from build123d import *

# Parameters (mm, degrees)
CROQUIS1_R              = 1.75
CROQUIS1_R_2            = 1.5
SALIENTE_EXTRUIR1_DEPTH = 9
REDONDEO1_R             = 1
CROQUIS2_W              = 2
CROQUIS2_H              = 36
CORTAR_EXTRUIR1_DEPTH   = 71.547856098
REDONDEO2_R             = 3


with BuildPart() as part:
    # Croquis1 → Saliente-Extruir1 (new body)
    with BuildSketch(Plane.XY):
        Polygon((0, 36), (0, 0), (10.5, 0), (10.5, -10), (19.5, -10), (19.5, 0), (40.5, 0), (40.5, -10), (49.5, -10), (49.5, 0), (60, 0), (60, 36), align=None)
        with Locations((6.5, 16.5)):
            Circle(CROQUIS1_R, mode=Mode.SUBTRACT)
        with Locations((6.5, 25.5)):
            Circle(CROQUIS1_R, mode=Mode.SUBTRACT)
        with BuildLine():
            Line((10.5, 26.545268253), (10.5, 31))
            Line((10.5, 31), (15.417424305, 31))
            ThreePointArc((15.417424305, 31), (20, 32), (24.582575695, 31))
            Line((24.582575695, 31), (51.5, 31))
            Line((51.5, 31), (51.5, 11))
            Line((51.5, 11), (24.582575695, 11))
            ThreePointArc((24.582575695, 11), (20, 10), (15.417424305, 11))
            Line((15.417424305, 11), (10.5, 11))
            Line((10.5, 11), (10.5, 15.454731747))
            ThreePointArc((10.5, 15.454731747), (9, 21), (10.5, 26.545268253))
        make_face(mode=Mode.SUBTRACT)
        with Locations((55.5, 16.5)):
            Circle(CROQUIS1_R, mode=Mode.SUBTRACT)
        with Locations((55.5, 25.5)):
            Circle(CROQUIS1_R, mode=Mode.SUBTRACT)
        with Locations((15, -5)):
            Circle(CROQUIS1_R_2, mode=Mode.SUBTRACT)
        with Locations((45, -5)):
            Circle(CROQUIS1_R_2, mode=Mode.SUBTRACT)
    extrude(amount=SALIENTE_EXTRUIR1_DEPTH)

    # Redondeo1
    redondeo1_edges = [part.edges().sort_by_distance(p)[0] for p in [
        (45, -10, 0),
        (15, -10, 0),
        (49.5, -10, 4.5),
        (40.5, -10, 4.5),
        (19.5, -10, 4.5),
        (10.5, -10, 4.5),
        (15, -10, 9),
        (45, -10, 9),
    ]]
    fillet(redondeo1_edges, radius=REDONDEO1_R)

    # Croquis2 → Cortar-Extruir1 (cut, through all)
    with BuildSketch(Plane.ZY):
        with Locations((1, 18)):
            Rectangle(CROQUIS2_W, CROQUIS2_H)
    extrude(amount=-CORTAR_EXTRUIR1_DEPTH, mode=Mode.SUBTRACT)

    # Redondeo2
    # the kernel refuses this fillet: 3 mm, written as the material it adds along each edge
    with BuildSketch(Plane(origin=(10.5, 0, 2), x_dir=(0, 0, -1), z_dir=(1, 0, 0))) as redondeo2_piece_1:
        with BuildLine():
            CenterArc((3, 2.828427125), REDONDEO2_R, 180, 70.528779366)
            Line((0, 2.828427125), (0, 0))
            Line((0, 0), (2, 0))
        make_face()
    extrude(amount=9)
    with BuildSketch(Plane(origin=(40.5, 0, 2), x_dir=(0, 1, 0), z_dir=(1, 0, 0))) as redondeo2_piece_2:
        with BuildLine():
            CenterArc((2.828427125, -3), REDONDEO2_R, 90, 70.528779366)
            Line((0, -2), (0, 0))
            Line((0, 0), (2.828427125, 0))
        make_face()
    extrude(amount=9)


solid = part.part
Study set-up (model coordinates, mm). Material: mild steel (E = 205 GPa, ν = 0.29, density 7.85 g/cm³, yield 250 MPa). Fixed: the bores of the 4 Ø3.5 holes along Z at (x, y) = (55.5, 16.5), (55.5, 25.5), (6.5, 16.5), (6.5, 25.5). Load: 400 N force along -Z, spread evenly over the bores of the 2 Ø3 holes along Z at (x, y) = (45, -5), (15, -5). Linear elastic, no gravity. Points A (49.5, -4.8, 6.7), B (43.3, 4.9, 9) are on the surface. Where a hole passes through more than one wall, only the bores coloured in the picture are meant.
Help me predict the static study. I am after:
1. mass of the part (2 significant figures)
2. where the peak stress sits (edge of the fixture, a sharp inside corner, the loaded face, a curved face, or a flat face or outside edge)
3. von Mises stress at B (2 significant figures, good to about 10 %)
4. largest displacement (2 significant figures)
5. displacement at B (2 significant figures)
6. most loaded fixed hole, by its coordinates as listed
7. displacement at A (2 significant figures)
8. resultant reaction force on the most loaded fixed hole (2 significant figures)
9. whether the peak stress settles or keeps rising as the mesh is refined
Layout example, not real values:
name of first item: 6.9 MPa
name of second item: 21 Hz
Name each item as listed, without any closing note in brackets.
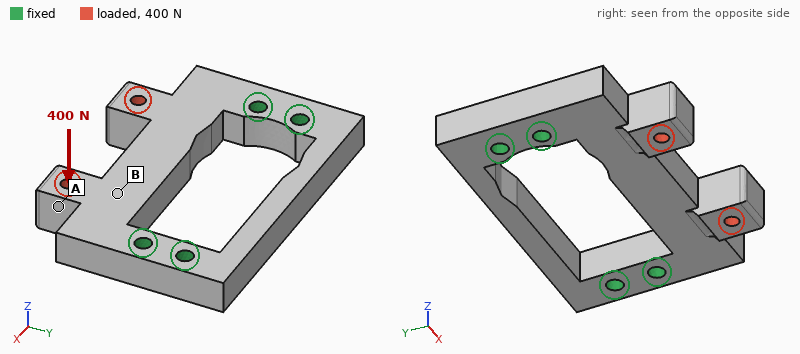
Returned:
mass of the part: 82 g
where the peak stress sits: edge of the fixture
von Mises stress at B: 14 MPa
largest displacement: 21 µm
displacement at B: 7.6 µm
most loaded fixed hole, by its coordinates as listed: (6.5, 16.5)
displacement at A: 14 µm
resultant reaction force on the most loaded fixed hole: 270 N
whether the peak stress settles or keeps rising as the mesh is refined: keeps rising
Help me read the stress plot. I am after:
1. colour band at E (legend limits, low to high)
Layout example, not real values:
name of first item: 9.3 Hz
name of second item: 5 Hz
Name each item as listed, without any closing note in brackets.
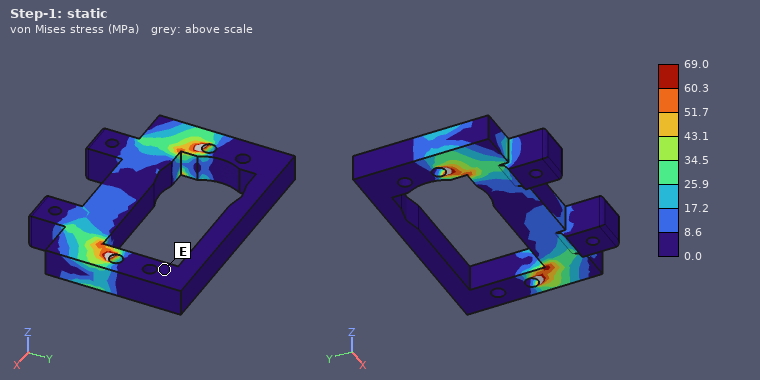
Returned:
colour band at E: 0.0 to 8.6 MPa
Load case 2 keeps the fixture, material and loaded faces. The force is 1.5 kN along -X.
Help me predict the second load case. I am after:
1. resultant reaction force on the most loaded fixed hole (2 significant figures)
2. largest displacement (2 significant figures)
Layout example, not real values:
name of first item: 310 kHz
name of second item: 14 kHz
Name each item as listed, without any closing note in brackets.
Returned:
resultant reaction force on the most loaded fixed hole: 990 N
largest displacement: 9.0 µm
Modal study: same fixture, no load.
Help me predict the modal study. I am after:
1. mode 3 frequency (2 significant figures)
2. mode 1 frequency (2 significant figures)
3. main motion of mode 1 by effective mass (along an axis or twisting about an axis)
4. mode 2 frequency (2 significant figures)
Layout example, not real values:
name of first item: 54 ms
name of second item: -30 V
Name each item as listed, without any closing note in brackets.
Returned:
mode 3 frequency: 11 kHz
mode 1 frequency: 5800 Hz
main motion of mode 1 by effective mass: along Z
mode 2 frequency: 10 kHz
